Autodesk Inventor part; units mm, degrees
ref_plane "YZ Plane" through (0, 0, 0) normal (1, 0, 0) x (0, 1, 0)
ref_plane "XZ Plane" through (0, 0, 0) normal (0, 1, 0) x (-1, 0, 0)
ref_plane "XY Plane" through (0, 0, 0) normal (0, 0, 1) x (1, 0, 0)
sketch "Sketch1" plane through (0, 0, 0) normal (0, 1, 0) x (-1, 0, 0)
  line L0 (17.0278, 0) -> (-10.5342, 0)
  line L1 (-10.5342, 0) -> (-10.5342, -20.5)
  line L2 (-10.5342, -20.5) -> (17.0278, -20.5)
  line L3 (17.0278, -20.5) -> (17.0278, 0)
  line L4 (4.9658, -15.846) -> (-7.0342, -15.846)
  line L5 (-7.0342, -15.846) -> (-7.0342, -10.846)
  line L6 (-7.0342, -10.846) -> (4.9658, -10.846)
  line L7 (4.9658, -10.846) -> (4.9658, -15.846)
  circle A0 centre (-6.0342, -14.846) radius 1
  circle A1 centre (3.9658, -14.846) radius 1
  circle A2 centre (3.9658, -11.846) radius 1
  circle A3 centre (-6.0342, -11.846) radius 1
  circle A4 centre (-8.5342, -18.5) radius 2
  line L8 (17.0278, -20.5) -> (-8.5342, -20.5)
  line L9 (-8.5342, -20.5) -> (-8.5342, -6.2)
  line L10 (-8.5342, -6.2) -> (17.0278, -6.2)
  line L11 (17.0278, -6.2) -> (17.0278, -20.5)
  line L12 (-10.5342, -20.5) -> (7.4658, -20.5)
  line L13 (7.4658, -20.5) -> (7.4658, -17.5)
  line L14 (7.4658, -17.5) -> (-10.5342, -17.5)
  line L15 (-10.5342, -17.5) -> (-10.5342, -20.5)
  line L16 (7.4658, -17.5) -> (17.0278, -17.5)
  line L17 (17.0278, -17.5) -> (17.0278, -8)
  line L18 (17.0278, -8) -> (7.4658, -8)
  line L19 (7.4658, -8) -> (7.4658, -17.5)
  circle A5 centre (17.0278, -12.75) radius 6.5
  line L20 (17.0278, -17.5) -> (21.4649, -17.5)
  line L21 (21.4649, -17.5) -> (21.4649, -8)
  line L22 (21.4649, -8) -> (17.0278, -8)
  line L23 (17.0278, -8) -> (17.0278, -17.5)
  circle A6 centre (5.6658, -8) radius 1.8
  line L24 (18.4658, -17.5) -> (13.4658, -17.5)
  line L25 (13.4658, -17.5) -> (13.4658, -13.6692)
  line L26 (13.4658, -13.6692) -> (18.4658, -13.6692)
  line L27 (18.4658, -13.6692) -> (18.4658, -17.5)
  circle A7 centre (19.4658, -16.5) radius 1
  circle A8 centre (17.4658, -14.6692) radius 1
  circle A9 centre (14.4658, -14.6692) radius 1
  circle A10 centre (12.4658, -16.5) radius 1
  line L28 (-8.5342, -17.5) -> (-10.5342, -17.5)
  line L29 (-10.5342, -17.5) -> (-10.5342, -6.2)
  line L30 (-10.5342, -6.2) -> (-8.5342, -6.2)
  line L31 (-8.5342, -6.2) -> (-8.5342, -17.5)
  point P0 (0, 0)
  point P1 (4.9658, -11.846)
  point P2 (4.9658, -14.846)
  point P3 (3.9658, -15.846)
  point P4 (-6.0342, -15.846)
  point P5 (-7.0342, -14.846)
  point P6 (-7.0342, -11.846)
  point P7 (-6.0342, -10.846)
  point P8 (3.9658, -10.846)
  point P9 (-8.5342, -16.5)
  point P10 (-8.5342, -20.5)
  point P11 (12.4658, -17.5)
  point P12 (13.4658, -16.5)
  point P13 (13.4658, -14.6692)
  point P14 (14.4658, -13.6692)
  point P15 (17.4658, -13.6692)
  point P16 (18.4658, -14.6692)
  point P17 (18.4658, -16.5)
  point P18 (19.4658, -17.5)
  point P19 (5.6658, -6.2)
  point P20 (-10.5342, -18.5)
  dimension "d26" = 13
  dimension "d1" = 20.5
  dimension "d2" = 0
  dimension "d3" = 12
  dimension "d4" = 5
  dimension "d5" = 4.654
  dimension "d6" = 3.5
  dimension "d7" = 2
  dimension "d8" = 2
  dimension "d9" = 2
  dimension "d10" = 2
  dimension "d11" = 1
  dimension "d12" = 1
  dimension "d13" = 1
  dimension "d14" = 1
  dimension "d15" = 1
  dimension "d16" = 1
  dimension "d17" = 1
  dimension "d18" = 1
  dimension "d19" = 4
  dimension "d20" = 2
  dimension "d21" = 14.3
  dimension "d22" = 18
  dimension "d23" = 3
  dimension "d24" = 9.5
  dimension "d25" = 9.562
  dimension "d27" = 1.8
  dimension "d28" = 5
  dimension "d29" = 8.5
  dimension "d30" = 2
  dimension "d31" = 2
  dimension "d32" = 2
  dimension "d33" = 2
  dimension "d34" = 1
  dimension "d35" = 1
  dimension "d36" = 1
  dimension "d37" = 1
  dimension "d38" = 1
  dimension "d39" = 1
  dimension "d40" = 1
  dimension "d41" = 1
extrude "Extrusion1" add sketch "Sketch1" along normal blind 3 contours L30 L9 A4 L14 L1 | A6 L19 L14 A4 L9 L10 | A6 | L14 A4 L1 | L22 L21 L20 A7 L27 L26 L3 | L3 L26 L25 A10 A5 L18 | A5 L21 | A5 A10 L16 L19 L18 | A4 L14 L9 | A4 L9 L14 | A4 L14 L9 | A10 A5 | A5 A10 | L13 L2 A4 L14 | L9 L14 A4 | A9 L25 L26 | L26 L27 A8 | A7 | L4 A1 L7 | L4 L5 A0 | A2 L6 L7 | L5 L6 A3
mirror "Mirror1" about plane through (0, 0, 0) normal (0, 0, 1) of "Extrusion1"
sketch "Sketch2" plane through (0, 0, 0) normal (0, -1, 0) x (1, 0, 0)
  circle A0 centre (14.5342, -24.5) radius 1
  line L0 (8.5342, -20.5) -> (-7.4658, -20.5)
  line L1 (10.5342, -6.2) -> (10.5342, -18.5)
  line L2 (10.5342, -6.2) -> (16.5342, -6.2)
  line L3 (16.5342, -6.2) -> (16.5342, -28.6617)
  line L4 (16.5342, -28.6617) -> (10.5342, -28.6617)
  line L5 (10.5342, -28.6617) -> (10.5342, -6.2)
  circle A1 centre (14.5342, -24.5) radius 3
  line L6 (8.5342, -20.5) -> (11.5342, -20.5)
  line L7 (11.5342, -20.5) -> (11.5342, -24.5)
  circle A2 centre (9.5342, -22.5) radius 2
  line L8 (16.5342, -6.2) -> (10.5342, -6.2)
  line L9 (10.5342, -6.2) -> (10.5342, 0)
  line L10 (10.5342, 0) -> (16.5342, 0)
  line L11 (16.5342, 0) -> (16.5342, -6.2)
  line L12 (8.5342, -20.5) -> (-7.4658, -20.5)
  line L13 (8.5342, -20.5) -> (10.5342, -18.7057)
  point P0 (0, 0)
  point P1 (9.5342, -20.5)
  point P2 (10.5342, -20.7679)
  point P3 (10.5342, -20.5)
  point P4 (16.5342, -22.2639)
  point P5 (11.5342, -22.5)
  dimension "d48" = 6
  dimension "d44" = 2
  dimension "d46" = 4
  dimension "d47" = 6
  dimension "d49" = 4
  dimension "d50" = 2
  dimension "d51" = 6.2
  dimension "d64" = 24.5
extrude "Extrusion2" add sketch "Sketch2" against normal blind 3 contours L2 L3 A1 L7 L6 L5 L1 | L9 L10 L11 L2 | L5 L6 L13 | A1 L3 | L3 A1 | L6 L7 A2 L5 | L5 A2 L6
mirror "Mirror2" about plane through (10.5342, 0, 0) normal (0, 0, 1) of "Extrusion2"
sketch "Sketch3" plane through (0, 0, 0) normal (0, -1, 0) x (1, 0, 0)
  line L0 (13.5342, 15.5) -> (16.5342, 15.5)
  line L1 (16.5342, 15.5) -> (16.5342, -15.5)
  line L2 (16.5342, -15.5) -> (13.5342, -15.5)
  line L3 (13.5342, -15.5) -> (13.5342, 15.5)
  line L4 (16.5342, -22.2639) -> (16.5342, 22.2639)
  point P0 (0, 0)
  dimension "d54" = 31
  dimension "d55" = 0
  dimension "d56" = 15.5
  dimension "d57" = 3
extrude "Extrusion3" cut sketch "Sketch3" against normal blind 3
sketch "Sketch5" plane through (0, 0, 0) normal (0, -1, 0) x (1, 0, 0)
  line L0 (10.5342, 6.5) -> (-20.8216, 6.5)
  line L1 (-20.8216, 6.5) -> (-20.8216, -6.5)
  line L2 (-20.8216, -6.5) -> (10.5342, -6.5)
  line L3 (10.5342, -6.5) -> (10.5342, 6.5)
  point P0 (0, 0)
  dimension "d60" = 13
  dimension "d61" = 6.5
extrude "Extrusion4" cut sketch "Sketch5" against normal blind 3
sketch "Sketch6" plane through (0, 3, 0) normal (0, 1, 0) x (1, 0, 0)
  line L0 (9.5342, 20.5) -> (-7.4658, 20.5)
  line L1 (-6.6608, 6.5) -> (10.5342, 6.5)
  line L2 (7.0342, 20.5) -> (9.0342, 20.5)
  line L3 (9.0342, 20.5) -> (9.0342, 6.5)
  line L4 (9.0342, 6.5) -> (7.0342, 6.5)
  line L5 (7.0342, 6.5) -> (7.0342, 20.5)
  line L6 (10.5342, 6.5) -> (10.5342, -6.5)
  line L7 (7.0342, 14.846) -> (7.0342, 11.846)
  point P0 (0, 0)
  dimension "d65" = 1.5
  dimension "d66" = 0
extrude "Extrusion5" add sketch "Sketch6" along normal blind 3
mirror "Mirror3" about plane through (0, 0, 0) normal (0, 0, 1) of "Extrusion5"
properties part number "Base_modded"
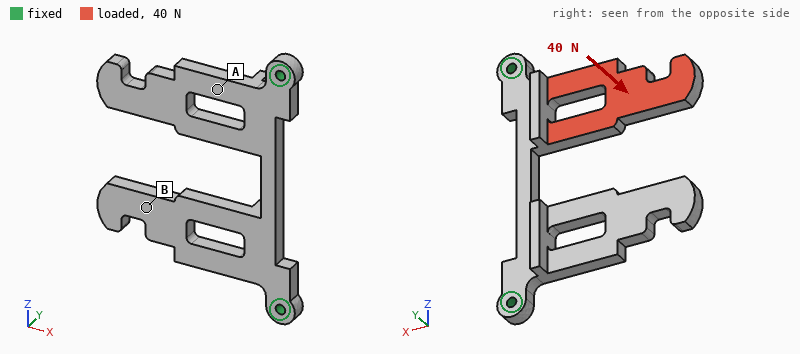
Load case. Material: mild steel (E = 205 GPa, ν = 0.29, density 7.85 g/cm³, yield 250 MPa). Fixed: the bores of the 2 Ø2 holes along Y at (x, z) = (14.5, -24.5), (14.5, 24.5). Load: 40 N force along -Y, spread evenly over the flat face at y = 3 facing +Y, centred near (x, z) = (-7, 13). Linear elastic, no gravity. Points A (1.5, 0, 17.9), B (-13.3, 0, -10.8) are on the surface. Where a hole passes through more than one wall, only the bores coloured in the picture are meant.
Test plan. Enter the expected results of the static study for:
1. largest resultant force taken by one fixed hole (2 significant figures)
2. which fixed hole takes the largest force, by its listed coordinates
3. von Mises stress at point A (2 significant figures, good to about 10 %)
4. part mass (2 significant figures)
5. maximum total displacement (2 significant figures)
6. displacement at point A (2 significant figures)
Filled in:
33 N
(14.5, 24.5)
31 MPa
22 g
0.13 mm
0.031 mm
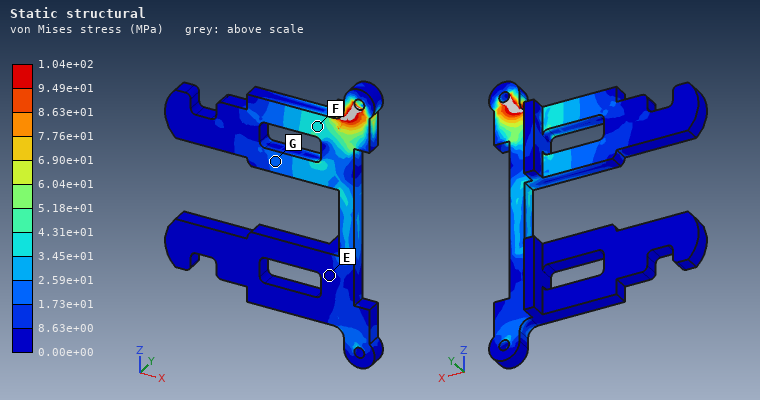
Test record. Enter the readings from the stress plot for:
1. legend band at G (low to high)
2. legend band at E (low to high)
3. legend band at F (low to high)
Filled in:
1.73e+01 to 2.59e+01 MPa
0.00e+00 to 8.63e+00 MPa
3.45e+01 to 4.31e+01 MPa
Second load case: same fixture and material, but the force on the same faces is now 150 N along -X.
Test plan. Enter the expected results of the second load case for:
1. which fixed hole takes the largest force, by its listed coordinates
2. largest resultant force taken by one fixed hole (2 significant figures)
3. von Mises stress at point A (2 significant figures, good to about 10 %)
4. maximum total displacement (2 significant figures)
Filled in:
(14.5, 24.5)
150 N
9.8 MPa
50 µm
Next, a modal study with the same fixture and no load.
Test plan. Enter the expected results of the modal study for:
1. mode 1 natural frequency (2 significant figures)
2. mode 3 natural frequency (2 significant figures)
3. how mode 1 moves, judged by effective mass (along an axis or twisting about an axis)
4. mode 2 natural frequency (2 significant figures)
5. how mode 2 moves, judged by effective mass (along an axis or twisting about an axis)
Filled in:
1300 Hz
2600 Hz
along Y
1500 Hz
twisting about X
